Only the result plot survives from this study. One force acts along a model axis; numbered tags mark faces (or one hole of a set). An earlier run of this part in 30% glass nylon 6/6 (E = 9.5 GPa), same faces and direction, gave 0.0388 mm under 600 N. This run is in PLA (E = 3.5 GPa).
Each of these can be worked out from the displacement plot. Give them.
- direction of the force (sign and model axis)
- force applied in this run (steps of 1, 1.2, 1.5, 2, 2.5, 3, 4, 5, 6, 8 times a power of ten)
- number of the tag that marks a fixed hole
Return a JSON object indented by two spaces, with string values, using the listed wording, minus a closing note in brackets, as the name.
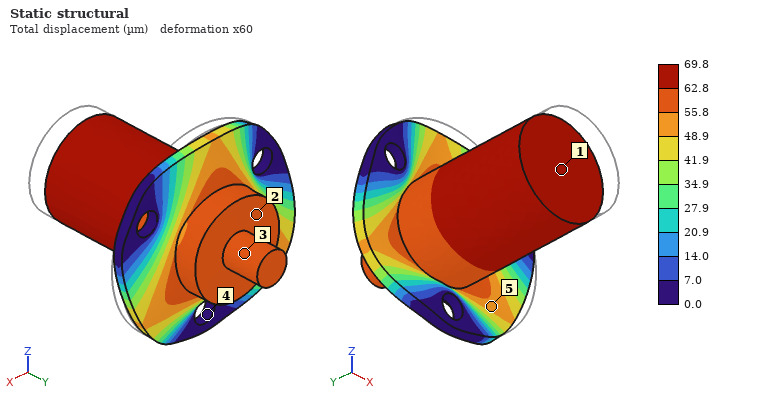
{
  "direction of the force": "+Y",
  "force applied in this run": "400 N",
  "number of the tag that marks a fixed hole": "4"
}
